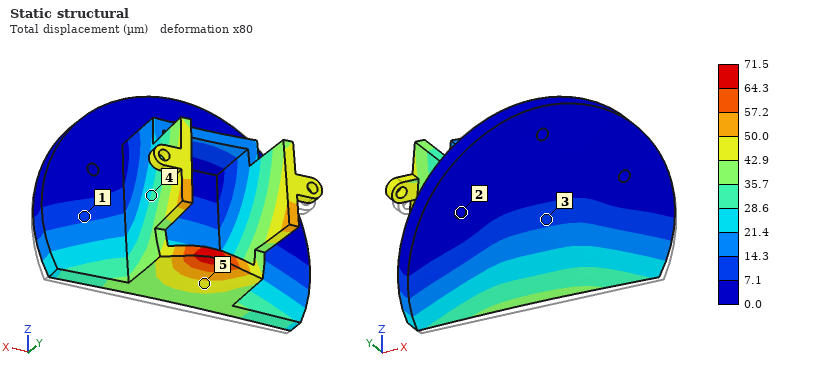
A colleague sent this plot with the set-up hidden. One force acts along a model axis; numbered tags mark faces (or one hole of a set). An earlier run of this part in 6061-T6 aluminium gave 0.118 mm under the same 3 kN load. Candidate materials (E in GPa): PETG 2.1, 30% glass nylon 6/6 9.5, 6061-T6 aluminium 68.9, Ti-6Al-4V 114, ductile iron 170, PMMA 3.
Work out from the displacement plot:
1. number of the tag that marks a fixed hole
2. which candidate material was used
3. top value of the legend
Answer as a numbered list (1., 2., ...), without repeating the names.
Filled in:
1. 2
2. Ti-6Al-4V
3. 71.5 µm
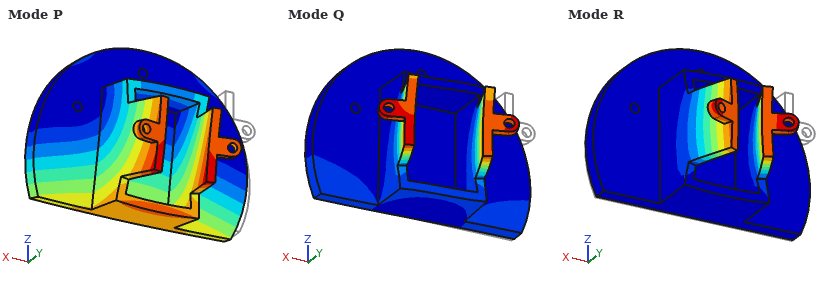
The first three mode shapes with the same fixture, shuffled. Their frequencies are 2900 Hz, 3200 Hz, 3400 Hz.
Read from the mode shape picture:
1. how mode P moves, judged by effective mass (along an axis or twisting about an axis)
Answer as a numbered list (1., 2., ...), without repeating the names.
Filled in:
1. along Y
